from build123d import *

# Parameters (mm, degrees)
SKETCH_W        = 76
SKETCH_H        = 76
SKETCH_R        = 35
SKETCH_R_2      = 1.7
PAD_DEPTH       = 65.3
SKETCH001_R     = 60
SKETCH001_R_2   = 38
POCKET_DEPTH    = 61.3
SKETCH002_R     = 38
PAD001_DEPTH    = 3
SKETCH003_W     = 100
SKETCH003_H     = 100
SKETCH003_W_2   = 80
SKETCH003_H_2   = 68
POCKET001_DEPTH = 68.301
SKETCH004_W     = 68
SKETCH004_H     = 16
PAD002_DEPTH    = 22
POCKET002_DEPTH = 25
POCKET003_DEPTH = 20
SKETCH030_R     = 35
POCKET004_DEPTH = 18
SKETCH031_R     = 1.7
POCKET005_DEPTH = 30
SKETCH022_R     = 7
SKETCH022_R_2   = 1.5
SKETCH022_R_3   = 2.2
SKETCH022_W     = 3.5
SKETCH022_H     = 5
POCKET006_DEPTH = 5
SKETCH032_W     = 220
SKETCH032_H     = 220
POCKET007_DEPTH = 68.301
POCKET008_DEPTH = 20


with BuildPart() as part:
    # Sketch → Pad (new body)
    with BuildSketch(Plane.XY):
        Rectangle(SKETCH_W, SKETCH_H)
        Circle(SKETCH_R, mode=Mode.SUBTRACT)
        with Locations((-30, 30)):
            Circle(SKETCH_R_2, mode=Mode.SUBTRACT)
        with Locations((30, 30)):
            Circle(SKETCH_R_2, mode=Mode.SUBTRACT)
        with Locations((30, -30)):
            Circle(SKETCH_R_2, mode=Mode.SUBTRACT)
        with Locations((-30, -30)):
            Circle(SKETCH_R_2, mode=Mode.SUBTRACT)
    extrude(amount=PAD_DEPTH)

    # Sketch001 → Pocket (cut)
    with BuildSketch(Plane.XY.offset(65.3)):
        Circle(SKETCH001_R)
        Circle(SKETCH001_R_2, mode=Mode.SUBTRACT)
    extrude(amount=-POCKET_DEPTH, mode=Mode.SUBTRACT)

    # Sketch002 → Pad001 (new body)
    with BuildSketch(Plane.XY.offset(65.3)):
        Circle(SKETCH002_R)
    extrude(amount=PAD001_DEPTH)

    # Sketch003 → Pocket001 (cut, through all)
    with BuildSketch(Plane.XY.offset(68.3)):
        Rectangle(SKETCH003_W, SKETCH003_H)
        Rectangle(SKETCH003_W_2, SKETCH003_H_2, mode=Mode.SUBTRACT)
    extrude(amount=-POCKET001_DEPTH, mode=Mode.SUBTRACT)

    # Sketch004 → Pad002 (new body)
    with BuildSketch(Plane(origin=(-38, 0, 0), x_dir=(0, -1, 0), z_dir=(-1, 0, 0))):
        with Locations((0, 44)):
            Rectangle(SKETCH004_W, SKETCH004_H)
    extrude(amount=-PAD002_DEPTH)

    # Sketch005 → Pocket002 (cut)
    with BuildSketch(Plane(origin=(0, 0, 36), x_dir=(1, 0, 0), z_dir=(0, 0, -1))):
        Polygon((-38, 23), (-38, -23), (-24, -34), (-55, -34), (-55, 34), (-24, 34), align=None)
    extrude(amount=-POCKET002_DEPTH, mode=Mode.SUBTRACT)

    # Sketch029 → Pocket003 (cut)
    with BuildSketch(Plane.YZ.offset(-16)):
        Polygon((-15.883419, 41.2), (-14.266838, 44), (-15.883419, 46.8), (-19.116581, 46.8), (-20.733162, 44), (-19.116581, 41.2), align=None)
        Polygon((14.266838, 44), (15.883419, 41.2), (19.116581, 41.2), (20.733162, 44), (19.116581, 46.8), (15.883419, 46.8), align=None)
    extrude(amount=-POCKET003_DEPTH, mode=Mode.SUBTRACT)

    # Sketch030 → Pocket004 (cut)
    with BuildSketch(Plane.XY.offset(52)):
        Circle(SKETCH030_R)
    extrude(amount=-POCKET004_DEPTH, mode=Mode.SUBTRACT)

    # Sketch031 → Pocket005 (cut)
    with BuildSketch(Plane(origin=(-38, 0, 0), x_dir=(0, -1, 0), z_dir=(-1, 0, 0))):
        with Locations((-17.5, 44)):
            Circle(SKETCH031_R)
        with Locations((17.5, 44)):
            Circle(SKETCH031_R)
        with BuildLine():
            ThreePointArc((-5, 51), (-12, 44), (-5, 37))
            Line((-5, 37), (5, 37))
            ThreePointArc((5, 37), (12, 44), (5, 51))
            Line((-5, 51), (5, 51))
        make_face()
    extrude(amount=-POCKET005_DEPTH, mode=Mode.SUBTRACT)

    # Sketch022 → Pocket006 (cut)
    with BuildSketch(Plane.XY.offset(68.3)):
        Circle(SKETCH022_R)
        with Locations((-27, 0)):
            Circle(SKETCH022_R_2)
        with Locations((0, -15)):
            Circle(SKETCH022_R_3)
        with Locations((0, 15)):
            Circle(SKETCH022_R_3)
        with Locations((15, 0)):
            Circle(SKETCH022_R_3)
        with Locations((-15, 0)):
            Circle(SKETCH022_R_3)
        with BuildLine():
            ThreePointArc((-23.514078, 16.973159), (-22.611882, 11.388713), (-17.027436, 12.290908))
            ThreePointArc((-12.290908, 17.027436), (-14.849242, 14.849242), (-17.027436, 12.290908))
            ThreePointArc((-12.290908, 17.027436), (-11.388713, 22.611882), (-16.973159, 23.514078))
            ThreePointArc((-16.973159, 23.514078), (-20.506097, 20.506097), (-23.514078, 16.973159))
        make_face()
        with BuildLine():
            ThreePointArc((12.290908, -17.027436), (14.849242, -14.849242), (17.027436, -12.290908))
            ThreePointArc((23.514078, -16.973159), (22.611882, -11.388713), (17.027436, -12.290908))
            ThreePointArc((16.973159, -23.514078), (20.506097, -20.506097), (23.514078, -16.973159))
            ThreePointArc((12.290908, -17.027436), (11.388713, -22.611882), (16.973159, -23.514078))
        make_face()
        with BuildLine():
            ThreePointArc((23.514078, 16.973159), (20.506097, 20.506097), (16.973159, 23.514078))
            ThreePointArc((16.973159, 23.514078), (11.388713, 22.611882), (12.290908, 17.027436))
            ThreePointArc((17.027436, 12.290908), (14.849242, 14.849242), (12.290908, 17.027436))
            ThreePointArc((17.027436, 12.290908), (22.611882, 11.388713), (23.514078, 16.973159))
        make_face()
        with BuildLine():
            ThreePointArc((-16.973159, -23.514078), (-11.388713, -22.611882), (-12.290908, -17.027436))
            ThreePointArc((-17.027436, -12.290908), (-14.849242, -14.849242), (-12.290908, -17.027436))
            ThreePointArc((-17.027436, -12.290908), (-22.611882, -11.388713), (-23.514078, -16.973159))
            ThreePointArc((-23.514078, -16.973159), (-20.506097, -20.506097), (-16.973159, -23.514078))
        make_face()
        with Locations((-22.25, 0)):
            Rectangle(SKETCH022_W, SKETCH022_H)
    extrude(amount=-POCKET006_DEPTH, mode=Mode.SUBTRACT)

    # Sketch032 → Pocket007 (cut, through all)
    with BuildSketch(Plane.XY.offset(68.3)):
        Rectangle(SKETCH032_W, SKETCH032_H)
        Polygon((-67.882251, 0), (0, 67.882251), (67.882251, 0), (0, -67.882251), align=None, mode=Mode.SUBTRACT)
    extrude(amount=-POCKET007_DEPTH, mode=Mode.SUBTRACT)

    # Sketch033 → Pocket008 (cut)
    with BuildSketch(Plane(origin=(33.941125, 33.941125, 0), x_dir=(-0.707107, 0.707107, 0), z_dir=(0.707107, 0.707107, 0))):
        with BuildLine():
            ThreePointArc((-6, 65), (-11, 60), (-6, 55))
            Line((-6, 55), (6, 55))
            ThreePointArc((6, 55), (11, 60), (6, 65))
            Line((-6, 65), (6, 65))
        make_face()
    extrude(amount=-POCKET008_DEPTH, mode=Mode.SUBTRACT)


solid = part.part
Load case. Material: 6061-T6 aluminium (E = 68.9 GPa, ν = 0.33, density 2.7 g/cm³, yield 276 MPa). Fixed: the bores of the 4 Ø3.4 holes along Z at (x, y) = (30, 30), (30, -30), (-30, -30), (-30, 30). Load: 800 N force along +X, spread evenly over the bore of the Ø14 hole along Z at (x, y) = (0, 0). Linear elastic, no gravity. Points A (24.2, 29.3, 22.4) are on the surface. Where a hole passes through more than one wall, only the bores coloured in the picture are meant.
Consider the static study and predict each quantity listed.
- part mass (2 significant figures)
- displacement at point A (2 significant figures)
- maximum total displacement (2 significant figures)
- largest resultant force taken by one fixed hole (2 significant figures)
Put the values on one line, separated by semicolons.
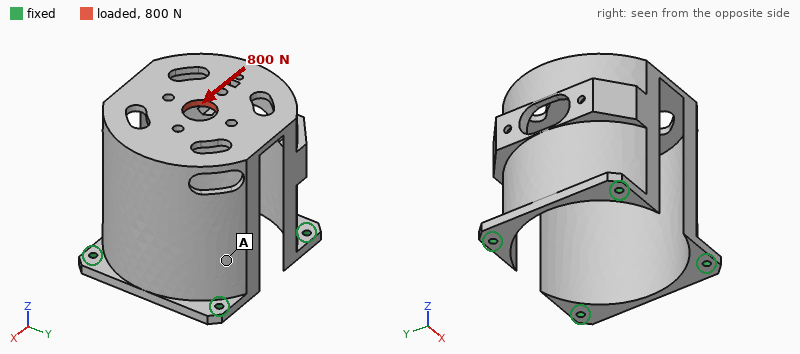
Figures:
140 g; 0.13 mm; 0.42 mm; 320 N
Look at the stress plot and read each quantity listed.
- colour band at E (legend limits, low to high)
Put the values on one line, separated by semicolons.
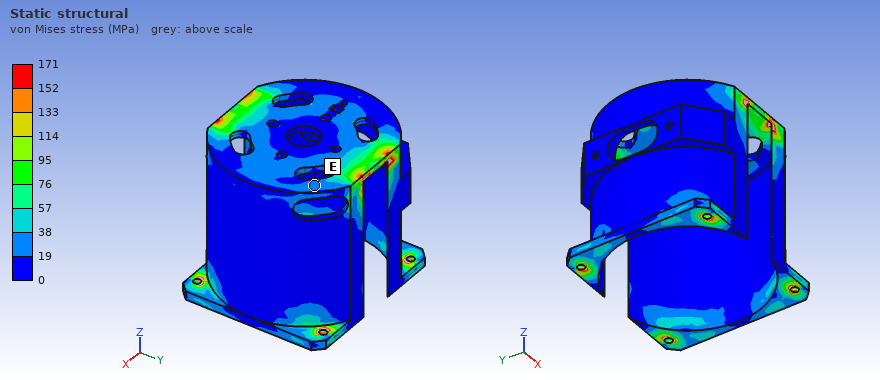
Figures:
19 to 38 MPa
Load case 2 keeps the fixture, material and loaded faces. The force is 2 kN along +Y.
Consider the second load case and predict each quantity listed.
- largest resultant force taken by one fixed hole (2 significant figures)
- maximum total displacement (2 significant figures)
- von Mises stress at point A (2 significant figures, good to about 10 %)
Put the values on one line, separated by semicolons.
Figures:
1.3 kN; 95 µm; 19 MPa
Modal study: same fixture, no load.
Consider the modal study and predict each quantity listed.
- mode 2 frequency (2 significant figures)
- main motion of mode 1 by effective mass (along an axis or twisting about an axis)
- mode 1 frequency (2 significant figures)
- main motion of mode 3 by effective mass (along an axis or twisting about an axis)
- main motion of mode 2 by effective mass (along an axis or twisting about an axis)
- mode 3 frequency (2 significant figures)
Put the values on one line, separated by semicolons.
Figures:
3100 Hz; along X; 890 Hz; along Y; along Y; 3400 Hz
